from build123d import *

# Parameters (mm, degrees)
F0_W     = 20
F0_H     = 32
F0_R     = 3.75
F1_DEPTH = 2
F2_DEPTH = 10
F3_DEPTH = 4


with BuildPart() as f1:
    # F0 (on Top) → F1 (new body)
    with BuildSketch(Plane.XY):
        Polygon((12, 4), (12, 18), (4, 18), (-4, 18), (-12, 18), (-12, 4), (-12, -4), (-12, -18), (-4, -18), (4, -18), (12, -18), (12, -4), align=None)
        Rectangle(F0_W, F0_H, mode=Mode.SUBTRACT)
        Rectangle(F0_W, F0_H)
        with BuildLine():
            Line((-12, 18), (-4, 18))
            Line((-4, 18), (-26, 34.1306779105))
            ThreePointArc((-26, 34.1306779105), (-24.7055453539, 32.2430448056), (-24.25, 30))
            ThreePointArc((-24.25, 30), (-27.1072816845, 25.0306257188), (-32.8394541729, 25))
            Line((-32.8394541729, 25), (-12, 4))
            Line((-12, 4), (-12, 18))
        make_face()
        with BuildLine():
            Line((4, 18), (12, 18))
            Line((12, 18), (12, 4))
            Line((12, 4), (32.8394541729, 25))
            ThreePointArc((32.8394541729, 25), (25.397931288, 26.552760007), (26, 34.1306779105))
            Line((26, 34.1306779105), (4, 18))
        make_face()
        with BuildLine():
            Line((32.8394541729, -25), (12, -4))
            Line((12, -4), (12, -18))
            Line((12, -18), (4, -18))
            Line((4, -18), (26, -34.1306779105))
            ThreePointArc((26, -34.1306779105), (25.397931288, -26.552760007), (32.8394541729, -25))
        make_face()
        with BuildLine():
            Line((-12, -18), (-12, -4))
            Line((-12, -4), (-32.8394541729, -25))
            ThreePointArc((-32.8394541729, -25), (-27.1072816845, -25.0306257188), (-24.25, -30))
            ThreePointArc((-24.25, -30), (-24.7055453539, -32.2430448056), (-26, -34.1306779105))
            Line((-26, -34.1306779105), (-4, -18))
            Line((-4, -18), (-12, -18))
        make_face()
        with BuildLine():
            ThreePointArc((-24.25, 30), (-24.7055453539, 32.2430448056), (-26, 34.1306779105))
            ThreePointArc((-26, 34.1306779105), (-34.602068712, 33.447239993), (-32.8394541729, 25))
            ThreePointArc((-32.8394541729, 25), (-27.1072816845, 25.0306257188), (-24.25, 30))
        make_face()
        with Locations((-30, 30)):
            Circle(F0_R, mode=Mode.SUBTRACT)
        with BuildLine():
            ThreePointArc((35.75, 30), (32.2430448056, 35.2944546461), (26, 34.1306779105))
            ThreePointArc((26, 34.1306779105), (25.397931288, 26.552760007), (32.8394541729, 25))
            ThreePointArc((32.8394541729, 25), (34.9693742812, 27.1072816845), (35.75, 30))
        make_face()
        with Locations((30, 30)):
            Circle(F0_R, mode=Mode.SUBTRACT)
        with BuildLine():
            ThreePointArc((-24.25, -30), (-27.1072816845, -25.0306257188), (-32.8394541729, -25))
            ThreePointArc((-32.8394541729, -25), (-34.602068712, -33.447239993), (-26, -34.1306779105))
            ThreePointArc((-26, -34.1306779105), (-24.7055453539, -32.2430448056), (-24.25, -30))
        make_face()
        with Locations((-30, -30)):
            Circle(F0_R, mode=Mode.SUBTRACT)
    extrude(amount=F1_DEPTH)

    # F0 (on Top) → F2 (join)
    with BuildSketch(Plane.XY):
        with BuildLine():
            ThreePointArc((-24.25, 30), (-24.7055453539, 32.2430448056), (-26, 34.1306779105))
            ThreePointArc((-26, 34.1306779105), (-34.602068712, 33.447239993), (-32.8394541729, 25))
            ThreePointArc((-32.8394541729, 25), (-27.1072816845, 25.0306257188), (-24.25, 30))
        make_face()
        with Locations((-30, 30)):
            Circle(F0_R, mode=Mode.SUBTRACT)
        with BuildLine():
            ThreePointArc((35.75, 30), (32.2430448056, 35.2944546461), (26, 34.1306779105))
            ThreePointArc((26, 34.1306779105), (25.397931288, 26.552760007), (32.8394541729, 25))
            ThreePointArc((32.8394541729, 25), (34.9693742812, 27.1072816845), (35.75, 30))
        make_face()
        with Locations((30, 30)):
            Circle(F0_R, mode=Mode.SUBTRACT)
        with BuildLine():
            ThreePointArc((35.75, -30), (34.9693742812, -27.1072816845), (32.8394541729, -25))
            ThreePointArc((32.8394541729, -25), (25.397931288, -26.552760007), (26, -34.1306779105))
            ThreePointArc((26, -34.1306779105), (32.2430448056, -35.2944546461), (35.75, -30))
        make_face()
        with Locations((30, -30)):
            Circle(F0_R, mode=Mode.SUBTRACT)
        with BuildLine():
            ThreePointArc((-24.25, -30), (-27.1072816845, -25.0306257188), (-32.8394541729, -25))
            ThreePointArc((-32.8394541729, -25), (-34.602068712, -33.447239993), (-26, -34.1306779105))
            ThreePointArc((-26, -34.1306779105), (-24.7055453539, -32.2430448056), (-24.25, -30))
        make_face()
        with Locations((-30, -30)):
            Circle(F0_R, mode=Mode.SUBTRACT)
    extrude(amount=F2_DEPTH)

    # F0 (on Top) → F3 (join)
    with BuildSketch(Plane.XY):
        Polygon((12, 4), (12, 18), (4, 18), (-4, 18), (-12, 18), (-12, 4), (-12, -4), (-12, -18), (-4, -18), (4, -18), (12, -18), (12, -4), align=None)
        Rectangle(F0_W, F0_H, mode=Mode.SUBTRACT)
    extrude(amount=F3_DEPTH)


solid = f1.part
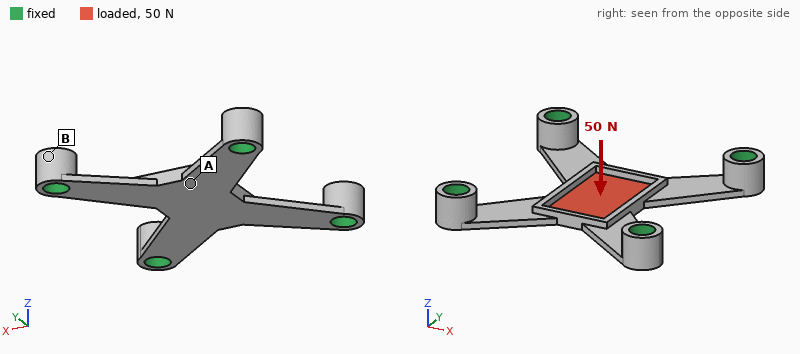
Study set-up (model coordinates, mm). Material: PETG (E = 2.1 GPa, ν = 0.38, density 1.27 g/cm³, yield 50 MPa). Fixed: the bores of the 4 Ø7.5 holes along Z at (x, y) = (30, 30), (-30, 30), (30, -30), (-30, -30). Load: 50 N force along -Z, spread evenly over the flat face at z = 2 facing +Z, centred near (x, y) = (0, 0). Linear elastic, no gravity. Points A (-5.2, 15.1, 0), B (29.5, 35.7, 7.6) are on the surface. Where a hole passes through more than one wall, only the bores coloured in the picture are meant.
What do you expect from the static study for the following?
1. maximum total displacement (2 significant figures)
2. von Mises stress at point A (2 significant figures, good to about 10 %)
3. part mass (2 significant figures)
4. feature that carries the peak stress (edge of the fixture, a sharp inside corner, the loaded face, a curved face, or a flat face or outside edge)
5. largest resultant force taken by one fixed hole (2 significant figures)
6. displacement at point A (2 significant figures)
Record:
1.1 mm
5.8 MPa
8.7 g
a flat face or outside edge
17 N
0.85 mm
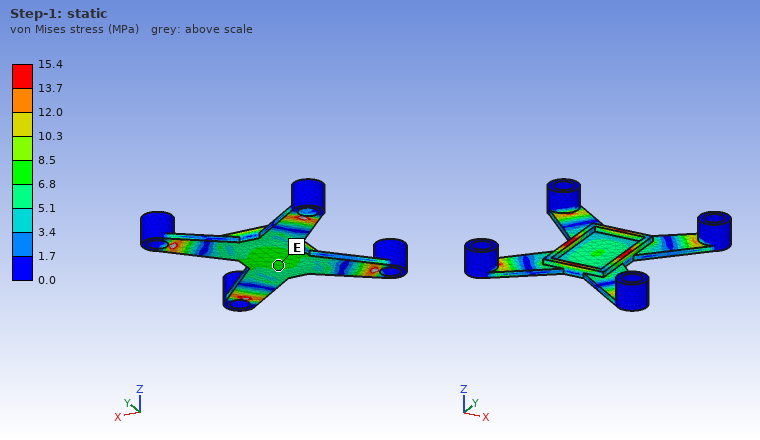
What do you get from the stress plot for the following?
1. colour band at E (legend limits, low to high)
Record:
6.8 to 8.5 MPa
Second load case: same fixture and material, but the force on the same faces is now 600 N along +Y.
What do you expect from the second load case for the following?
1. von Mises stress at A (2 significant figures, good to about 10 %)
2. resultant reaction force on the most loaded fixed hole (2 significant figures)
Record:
2.2 MPa
200 N
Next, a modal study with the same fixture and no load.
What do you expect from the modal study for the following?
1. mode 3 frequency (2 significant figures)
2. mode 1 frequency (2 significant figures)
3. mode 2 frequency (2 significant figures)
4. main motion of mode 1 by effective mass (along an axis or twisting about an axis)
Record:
1400 Hz
640 Hz
1300 Hz
along Z
